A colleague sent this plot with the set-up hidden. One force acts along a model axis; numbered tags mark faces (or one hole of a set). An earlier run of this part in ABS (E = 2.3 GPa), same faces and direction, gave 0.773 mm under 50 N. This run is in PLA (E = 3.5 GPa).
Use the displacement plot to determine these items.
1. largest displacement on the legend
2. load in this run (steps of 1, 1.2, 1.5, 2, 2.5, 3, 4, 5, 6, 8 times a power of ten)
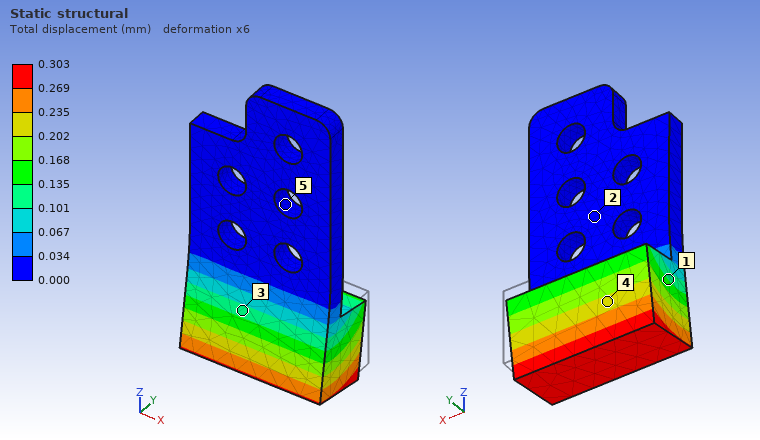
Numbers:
0.303 mm
30 N
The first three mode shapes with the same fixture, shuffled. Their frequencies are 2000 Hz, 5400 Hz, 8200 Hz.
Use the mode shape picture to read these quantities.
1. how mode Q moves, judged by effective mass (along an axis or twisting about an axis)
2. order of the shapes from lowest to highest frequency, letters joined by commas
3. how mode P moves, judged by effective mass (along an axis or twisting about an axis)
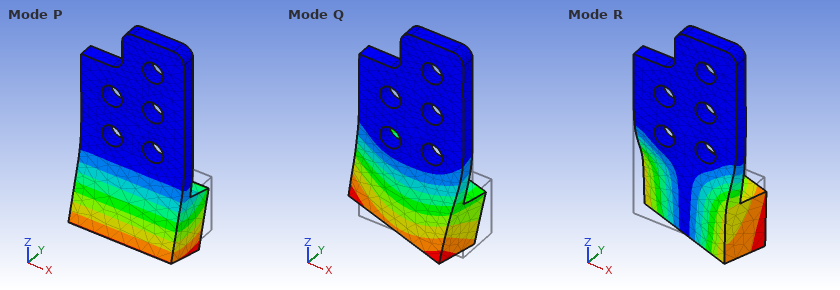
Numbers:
along X
P, R, Q
along Y
